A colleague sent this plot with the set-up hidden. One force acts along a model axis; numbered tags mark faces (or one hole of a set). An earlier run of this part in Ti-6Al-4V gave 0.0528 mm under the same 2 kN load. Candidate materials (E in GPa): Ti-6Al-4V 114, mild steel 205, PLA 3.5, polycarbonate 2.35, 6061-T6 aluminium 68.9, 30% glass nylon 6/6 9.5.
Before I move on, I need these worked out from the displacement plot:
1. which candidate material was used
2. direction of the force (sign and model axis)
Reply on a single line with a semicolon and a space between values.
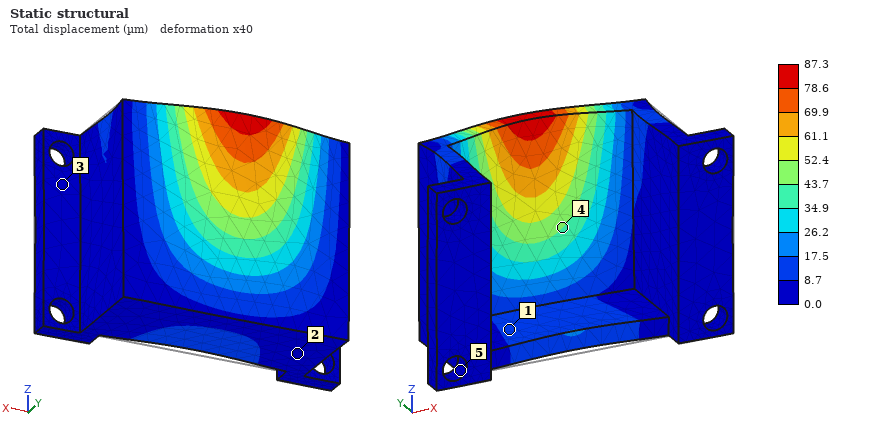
6061-T6 aluminium; +Y
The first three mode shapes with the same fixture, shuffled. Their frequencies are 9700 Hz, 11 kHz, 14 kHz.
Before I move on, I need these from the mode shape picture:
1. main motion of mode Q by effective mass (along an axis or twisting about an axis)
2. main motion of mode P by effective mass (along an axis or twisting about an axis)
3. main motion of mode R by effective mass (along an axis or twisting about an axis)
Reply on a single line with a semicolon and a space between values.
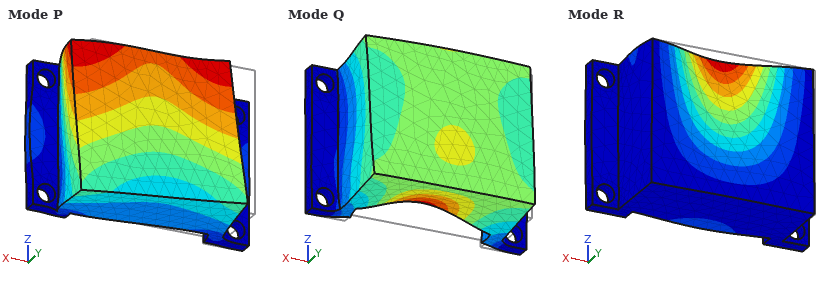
along Z; along X; along Y
